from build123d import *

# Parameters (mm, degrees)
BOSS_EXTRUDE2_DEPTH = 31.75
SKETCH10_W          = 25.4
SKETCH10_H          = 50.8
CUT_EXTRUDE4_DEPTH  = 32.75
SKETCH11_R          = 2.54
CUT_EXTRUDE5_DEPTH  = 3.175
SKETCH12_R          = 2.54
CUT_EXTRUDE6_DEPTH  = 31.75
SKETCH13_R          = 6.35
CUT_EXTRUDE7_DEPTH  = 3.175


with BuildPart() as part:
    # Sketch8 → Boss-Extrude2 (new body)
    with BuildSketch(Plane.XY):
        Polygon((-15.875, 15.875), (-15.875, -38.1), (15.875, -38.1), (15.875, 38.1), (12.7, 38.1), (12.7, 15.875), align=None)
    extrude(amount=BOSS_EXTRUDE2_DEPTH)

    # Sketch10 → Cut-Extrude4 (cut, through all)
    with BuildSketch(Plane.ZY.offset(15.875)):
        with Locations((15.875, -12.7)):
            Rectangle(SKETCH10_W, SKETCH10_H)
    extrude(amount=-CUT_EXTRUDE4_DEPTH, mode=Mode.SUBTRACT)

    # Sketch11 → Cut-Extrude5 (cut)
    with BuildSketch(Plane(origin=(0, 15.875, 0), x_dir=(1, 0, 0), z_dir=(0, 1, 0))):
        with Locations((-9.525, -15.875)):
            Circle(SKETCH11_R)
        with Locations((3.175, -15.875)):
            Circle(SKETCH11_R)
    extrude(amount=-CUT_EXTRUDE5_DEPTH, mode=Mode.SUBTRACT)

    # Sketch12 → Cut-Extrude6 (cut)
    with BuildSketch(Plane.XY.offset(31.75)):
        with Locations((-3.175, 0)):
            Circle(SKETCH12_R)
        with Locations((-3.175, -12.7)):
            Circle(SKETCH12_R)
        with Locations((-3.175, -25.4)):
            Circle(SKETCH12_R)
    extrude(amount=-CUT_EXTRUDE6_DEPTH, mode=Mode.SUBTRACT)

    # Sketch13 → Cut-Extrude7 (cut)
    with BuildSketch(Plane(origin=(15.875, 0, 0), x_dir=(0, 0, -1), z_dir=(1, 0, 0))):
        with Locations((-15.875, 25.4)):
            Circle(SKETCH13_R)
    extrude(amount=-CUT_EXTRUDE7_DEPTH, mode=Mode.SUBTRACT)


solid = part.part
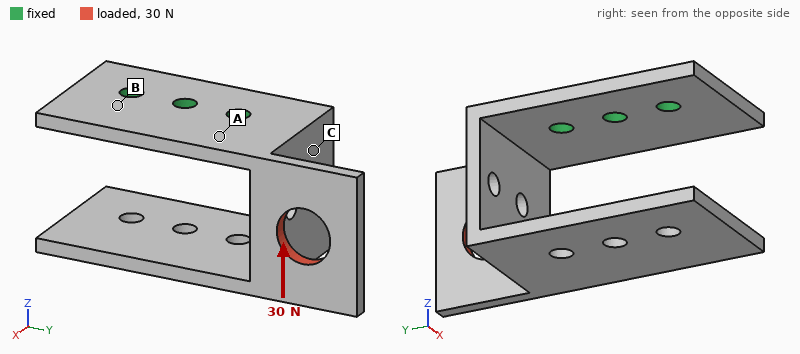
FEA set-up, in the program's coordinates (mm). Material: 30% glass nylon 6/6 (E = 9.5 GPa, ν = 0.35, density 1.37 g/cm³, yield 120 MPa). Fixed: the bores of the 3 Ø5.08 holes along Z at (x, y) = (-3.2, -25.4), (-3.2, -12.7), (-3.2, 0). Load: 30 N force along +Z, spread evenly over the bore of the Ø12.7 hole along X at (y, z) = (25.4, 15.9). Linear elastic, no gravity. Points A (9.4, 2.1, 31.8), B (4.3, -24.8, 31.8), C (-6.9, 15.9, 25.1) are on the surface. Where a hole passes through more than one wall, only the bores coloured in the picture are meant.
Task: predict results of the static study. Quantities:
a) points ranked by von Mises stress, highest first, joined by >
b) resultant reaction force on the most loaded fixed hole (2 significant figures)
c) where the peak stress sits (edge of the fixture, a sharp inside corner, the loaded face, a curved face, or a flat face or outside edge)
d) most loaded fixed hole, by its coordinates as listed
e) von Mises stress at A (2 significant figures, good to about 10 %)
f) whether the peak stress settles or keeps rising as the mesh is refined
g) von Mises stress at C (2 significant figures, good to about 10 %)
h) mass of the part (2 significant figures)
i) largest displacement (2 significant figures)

A > C > B
49 N
edge of the fixture
(-3.2, 0)
10 MPa
keeps rising
5.7 MPa
20 g
0.84 mm
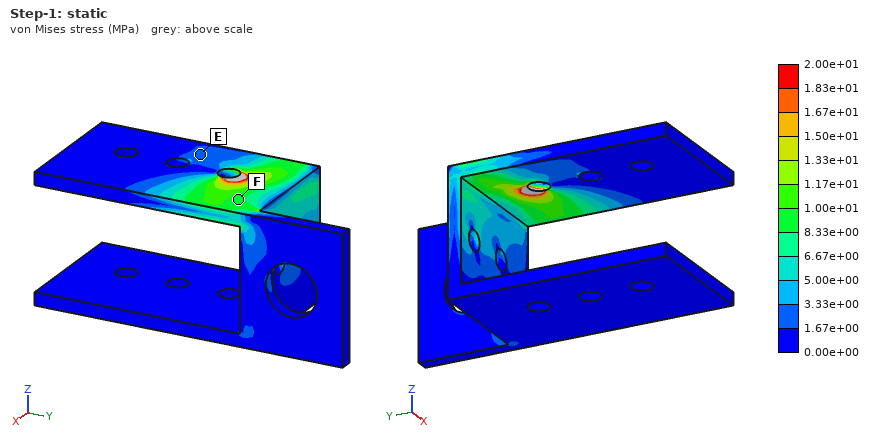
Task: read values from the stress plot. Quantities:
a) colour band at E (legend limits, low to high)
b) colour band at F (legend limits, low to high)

1.67e+00 to 3.33e+00 MPa
8.33e+00 to 1.00e+01 MPa
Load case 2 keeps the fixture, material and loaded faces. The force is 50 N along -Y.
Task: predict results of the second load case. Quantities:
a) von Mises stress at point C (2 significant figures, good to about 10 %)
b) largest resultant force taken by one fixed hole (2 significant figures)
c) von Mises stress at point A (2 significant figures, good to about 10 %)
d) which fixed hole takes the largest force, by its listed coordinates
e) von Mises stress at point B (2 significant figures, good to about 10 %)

7.9 MPa
46 N
9.0 MPa
(-3.2, 0)
1.6 MPa
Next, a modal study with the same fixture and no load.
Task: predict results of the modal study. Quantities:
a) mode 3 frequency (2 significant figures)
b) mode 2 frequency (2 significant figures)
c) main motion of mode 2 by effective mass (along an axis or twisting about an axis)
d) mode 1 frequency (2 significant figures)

590 Hz
350 Hz
along X
250 Hz
